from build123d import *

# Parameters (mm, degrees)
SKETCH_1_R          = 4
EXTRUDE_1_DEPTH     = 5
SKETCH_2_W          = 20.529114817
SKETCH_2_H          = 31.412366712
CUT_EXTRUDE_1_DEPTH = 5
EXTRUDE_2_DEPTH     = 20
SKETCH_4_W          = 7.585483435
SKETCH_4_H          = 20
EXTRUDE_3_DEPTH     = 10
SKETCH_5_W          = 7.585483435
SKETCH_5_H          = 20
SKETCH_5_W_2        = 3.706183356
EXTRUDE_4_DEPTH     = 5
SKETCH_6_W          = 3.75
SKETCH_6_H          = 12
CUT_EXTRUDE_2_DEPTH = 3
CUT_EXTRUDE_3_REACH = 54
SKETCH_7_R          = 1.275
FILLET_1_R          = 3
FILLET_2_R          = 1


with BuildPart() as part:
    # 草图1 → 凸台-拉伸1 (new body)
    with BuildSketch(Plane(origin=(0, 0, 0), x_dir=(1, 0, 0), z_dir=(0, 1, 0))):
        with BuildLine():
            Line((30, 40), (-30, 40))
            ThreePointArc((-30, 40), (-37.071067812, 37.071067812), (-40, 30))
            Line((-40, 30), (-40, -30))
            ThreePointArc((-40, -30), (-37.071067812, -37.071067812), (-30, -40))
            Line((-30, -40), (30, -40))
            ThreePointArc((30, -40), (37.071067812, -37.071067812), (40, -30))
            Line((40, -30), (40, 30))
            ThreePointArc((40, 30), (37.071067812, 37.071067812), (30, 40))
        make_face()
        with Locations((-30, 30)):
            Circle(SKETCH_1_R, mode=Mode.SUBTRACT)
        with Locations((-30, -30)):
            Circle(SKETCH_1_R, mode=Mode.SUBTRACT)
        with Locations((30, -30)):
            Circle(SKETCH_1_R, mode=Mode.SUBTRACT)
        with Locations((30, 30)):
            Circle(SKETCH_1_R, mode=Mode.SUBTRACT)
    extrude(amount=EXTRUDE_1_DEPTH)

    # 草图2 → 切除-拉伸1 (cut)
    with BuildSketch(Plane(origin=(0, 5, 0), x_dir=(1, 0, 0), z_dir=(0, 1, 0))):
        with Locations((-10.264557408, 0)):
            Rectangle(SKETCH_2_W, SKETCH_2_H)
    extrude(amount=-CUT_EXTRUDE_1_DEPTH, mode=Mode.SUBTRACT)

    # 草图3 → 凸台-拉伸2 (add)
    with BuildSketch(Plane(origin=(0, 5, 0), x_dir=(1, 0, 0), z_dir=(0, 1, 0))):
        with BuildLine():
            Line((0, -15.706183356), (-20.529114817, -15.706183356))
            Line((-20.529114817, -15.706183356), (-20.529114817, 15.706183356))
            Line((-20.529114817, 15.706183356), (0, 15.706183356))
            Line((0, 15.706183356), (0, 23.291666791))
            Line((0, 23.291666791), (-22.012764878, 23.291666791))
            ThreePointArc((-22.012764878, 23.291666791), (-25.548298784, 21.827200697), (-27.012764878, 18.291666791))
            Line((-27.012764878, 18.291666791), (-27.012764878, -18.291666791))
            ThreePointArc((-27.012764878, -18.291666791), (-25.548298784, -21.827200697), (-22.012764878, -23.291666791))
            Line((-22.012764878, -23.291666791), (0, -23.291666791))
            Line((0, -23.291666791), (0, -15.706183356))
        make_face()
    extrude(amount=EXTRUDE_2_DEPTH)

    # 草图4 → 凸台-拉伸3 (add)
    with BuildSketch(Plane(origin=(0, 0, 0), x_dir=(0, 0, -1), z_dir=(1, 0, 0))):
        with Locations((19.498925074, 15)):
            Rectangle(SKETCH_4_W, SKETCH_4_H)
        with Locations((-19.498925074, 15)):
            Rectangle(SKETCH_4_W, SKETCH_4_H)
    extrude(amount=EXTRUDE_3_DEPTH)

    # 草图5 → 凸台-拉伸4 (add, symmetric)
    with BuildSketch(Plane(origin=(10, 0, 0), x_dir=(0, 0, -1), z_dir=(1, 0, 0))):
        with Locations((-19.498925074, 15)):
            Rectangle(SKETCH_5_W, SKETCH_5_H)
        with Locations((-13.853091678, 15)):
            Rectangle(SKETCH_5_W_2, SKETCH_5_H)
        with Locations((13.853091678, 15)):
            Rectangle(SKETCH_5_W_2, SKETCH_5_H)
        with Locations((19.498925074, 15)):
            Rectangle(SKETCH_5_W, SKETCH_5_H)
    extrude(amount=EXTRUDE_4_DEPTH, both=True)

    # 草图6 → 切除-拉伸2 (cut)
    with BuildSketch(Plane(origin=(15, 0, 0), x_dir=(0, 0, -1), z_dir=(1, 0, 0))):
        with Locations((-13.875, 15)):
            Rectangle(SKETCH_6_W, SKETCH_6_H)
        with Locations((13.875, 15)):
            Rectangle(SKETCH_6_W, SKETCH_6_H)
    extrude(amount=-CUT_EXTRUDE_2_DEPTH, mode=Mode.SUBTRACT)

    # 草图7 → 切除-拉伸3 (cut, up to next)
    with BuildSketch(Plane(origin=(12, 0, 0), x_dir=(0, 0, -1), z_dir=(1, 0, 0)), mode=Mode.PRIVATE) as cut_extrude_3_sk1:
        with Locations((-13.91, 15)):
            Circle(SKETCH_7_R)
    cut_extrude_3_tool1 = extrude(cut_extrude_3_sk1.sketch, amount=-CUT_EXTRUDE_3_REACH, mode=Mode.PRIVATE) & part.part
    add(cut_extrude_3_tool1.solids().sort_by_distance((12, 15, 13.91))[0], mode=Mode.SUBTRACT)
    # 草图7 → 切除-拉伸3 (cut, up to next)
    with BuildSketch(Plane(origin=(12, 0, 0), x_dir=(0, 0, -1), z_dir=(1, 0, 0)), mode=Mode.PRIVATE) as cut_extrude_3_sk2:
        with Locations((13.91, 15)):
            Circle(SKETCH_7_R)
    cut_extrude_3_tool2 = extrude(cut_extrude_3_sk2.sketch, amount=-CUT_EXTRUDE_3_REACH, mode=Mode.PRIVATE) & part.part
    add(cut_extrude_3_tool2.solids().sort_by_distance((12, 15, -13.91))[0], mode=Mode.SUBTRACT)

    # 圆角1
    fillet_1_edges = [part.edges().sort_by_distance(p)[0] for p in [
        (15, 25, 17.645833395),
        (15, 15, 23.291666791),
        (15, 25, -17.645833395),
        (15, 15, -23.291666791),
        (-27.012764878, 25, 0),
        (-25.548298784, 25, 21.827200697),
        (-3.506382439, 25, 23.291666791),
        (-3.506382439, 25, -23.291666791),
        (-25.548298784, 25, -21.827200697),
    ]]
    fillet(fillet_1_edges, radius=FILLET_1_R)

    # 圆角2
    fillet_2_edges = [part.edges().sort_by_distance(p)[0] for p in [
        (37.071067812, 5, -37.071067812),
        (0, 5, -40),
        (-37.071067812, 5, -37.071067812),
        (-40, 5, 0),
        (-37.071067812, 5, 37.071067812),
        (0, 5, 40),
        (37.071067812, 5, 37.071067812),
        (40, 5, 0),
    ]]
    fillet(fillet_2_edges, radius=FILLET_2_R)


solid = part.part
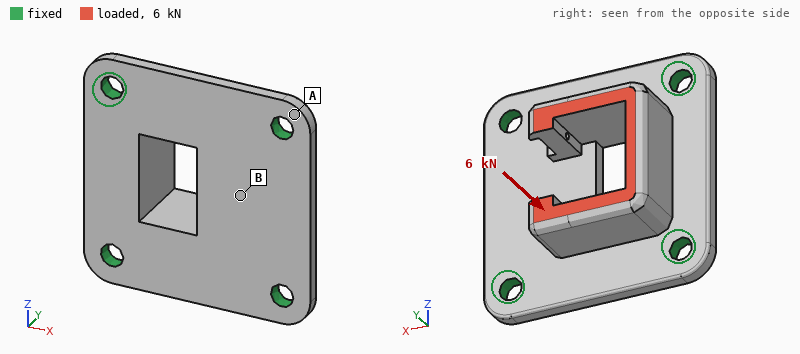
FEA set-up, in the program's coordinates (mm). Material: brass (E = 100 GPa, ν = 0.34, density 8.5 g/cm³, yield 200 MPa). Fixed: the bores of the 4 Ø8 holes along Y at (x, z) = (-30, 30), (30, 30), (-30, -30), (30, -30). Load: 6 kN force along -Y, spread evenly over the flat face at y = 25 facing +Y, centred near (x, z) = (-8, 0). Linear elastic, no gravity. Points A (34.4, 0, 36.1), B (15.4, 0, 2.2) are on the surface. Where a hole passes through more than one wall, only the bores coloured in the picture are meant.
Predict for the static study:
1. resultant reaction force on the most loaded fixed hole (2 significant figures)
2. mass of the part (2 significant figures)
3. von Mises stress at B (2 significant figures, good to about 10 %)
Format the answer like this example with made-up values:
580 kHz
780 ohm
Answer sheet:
2.2 kN
380 g
26 MPa
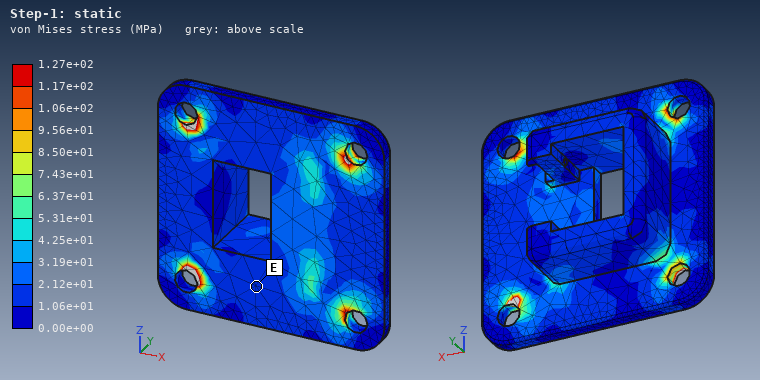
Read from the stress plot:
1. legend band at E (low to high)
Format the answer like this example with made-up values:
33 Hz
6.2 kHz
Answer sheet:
1.06e+01 to 2.12e+01 MPa
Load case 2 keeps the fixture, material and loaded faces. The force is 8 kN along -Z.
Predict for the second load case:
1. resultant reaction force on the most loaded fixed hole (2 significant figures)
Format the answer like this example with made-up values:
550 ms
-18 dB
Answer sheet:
3.9 kN
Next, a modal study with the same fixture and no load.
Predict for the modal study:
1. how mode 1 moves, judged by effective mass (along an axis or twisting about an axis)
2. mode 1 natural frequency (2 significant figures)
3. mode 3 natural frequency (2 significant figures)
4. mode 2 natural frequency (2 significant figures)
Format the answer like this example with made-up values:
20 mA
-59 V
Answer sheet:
along Y
4000 Hz
5800 Hz
5600 Hz
